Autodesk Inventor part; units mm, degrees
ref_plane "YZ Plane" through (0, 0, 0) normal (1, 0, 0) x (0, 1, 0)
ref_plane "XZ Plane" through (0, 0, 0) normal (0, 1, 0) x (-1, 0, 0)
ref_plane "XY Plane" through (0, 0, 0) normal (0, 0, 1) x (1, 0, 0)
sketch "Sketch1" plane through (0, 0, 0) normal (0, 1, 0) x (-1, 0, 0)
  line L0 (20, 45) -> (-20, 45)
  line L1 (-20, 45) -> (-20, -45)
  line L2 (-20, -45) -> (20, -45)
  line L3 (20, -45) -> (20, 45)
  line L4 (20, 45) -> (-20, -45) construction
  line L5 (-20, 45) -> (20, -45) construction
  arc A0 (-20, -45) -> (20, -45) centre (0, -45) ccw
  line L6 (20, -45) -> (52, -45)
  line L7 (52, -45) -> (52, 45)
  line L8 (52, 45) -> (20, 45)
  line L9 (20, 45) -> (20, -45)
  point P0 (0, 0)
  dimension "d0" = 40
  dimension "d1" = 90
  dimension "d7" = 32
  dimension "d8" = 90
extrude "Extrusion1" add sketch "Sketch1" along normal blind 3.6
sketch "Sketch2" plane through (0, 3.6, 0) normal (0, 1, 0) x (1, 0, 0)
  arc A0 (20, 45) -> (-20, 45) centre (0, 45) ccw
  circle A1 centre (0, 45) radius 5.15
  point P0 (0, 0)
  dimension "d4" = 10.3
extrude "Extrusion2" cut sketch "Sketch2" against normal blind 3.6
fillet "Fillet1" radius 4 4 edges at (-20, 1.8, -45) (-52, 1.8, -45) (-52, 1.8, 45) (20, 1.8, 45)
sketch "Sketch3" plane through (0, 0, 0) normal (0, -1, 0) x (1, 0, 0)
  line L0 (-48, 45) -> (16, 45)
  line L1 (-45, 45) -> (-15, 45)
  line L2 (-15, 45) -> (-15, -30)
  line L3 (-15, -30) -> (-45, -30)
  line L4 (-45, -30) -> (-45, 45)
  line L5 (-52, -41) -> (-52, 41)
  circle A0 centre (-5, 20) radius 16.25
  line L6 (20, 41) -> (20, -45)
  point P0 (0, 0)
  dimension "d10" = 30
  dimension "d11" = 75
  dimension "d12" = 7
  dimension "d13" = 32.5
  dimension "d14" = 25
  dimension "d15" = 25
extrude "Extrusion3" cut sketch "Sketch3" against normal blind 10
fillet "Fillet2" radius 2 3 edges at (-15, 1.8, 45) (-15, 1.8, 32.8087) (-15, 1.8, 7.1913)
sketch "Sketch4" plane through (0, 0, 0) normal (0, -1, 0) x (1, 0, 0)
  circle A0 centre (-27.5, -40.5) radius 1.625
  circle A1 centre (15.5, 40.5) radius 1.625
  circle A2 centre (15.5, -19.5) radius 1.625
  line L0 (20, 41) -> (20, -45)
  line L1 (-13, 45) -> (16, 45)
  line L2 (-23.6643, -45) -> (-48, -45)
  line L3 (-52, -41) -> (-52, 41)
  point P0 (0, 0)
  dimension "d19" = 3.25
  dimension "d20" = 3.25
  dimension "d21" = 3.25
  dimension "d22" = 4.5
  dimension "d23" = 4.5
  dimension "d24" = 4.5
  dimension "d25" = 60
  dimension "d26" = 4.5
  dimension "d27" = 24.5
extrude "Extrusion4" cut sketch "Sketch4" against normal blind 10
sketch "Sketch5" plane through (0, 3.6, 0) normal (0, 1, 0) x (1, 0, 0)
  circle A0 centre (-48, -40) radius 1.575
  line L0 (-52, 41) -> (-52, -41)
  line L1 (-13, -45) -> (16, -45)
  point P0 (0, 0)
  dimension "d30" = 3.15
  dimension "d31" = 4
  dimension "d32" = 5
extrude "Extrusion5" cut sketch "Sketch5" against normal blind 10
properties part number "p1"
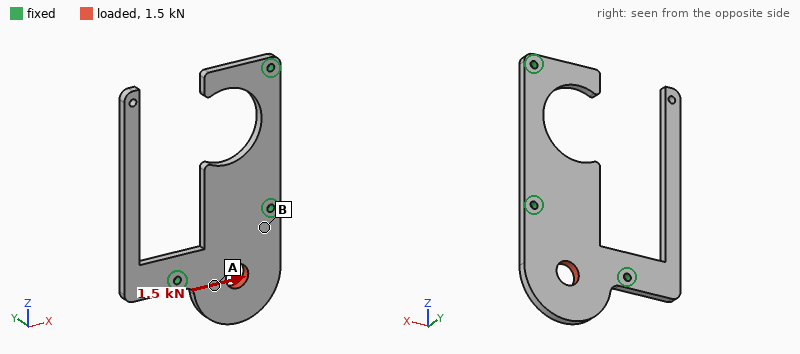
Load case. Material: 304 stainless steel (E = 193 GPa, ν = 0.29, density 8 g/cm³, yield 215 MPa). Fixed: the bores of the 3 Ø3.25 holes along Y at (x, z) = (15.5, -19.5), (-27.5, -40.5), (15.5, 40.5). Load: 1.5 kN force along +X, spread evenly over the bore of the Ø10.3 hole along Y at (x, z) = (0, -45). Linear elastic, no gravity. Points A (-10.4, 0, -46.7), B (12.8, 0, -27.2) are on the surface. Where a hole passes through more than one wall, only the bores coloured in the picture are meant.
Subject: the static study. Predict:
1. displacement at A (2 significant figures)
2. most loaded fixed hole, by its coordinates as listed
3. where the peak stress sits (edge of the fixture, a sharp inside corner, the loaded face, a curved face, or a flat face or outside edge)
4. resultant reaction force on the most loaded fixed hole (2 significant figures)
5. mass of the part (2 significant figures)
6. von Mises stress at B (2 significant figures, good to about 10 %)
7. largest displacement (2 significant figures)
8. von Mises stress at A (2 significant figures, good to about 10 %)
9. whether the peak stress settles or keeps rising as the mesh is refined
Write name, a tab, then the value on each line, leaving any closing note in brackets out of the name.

displacement at A	2.8 µm
most loaded fixed hole, by its coordinates as listed	(-27.5, -40.5)
where the peak stress sits	edge of the fixture
resultant reaction force on the most loaded fixed hole	1.1 kN
mass of the part	120 g
von Mises stress at B	11 MPa
largest displacement	12 µm
von Mises stress at A	24 MPa
whether the peak stress settles or keeps rising as the mesh is refined	keeps rising
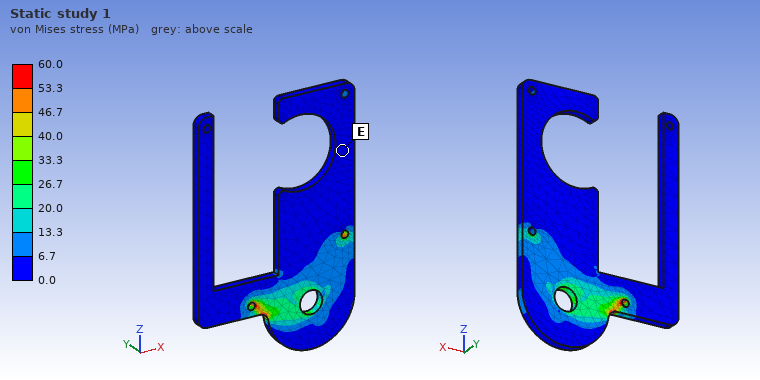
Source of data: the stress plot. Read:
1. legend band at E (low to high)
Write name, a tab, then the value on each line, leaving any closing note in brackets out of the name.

legend band at E	0.0 to 6.7 MPa
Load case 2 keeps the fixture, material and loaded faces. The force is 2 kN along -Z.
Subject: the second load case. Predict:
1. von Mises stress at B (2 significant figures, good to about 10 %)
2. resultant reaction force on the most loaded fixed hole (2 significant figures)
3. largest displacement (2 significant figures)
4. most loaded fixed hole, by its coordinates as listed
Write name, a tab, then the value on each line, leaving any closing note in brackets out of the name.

von Mises stress at B	27 MPa
resultant reaction force on the most loaded fixed hole	1.4 kN
largest displacement	16 µm
most loaded fixed hole, by its coordinates as listed	(15.5, -19.5)
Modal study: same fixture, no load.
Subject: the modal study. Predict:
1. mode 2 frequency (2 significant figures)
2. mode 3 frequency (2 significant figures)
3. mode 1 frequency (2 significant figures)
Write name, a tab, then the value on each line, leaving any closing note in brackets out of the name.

mode 2 frequency	860 Hz
mode 3 frequency	2000 Hz
mode 1 frequency	390 Hz
